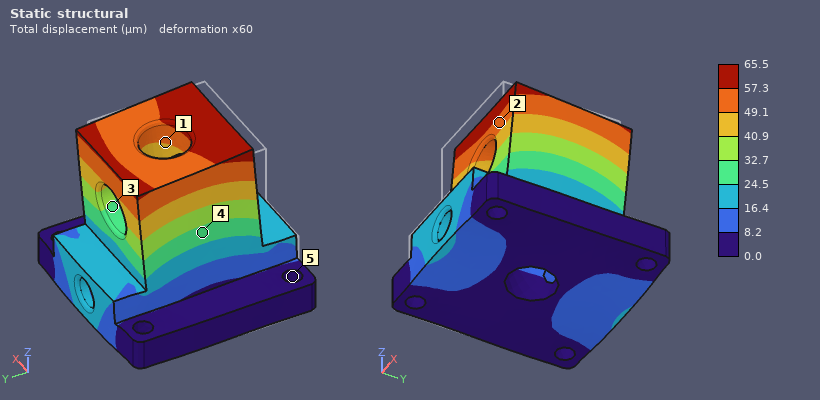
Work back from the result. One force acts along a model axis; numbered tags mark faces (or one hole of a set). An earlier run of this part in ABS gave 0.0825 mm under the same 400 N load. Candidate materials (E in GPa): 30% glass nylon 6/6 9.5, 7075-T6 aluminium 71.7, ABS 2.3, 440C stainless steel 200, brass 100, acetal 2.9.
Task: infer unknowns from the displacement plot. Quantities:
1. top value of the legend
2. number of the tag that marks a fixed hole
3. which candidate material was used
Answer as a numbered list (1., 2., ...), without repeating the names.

1. 65.5 µm
2. 5
3. acetal
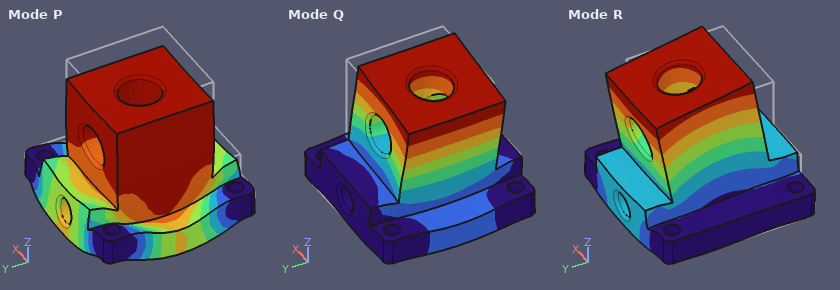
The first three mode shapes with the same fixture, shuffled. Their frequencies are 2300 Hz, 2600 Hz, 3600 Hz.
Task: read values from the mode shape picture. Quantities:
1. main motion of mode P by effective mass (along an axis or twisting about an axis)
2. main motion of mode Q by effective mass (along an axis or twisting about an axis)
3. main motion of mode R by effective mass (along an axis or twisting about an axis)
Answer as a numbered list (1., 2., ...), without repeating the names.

1. along Z
2. along X
3. along Y
